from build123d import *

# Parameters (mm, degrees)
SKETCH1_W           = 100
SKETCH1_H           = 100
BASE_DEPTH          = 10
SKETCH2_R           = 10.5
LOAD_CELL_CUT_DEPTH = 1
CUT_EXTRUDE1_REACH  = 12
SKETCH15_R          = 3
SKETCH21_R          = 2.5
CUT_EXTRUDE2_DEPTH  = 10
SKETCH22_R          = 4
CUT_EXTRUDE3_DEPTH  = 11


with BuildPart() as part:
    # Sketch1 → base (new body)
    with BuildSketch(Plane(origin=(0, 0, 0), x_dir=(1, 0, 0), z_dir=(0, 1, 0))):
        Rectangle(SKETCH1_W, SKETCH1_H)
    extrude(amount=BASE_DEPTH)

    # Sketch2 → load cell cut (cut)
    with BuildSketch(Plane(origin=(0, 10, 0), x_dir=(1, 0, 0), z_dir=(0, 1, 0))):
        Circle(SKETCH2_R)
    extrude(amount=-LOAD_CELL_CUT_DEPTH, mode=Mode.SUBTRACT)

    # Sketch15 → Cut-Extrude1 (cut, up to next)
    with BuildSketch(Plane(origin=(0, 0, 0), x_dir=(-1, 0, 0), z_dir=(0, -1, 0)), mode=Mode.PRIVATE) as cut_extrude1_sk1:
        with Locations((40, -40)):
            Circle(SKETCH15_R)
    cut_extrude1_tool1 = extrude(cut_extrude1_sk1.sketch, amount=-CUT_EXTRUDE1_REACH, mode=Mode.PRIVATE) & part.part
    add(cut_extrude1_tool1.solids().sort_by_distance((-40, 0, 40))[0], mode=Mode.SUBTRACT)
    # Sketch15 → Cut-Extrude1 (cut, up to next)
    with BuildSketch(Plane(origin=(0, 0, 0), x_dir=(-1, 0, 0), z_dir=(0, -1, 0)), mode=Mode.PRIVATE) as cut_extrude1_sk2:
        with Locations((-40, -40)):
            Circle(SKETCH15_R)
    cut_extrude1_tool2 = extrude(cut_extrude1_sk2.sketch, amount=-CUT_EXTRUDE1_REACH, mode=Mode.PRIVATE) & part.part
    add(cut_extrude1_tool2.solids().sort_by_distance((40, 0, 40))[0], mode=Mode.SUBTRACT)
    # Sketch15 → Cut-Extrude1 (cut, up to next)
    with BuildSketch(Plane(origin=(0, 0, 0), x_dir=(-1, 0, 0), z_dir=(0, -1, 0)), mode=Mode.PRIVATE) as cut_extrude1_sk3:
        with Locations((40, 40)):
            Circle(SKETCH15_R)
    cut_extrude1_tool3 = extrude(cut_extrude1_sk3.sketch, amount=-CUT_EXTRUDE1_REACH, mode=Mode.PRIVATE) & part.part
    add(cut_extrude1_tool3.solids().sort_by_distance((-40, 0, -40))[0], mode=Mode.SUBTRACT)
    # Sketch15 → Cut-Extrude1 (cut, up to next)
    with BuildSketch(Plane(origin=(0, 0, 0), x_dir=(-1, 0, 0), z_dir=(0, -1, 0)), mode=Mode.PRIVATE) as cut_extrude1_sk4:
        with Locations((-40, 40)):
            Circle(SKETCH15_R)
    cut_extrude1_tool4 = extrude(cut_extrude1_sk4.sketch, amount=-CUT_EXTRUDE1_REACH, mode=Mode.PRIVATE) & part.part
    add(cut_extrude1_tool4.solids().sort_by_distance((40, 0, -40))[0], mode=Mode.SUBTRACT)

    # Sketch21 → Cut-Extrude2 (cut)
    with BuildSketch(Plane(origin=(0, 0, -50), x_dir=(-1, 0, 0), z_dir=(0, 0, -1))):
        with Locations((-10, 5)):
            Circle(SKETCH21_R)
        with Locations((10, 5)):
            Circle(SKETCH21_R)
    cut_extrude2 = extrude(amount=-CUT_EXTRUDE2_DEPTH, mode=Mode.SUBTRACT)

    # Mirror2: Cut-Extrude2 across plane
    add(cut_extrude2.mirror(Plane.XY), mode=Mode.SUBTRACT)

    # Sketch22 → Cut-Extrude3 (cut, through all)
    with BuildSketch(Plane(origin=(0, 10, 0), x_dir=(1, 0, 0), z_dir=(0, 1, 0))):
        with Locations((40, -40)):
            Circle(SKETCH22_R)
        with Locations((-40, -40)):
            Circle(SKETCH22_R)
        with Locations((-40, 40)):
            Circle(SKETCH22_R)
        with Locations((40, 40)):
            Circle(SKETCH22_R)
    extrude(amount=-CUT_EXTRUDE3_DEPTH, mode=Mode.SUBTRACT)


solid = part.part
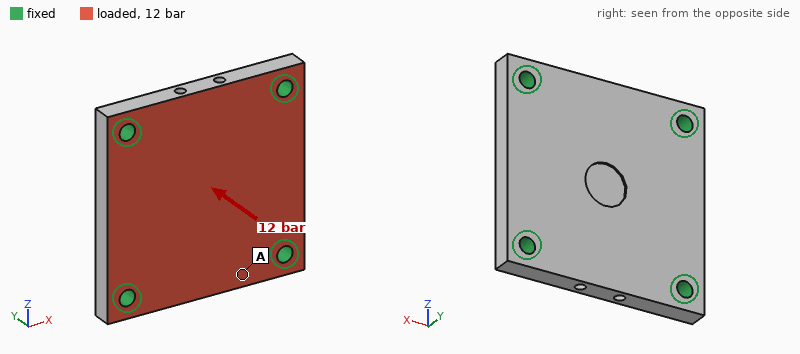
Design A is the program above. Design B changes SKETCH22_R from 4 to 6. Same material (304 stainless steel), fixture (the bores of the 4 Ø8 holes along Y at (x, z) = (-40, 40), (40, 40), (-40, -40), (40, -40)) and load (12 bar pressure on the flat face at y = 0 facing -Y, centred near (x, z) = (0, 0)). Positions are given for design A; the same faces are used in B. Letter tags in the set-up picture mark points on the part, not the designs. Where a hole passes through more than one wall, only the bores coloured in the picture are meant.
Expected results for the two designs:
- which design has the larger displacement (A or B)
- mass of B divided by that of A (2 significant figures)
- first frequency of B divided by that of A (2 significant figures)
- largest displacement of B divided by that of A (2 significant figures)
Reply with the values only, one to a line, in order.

A
0.97
1.1
0.80
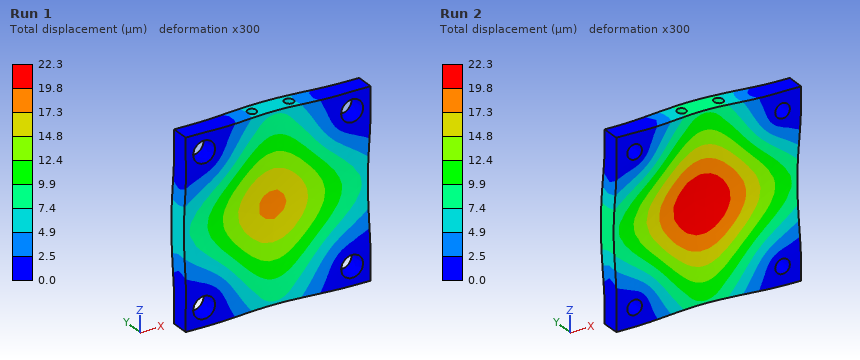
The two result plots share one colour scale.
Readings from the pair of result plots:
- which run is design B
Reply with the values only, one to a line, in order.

Run 1
